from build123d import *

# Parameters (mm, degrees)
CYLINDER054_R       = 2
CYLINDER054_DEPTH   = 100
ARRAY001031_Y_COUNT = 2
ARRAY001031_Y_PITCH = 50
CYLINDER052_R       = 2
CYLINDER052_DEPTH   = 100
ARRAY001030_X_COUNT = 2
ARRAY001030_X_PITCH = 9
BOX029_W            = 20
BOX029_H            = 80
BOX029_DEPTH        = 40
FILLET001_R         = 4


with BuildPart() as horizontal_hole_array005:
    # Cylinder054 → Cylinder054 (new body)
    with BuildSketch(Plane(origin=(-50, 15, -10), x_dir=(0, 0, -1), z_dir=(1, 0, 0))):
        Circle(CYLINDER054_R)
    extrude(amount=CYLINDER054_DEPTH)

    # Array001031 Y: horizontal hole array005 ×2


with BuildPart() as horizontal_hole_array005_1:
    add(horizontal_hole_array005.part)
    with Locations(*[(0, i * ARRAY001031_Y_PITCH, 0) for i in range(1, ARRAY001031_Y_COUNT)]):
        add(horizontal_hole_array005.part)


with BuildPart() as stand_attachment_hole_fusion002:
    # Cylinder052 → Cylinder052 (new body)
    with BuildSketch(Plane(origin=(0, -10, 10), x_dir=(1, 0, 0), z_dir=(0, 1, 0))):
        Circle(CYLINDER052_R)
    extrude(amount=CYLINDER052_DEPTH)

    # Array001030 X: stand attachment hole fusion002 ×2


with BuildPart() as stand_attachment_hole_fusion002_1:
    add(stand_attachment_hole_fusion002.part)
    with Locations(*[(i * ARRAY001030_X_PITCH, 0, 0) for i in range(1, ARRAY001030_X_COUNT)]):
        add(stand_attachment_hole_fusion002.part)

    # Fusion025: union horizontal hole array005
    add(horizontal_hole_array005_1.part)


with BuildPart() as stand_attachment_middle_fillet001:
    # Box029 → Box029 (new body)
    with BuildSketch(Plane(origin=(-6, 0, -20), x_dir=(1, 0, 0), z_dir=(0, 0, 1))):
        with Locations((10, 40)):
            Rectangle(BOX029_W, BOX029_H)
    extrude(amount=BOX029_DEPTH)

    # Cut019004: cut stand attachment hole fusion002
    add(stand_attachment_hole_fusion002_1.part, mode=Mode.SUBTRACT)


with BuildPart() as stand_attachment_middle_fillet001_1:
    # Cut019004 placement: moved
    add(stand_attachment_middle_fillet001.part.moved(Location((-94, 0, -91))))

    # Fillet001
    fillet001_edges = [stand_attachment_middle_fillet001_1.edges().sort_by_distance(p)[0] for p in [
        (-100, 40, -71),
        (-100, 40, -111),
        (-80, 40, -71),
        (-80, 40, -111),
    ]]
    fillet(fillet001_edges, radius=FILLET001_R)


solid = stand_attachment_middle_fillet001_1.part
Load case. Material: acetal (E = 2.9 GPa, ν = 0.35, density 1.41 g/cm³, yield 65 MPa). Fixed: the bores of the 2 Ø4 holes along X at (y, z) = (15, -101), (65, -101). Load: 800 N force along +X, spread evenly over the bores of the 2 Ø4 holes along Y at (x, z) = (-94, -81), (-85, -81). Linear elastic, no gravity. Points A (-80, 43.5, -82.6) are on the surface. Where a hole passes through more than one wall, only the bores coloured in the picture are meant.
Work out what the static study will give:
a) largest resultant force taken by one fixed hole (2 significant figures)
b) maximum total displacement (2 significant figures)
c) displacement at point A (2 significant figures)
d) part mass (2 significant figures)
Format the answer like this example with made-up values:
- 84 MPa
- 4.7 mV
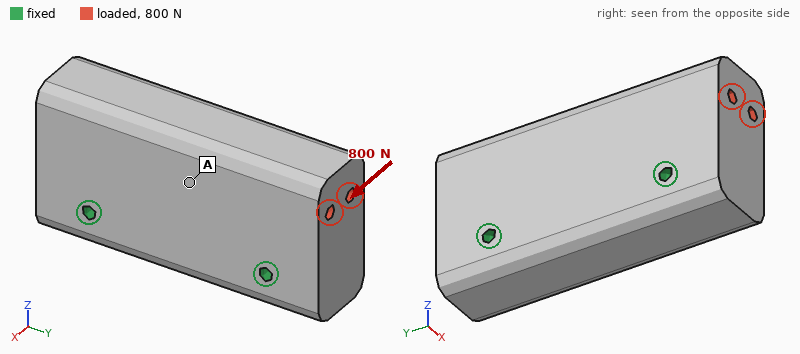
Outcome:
- 400 N
- 84 µm
- 59 µm
- 85 g
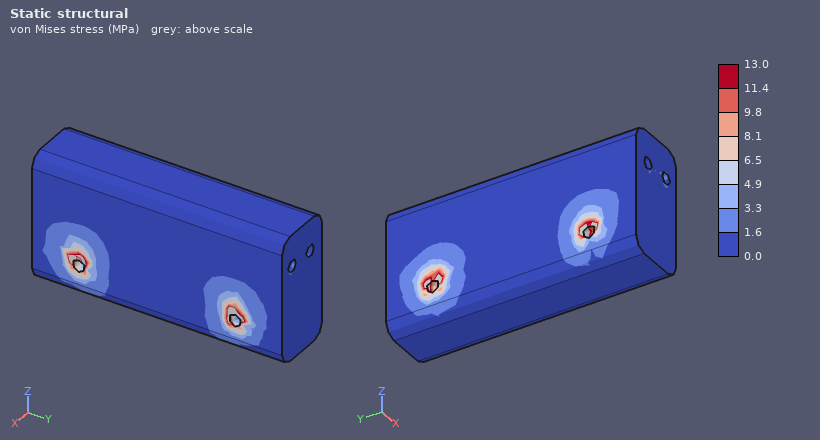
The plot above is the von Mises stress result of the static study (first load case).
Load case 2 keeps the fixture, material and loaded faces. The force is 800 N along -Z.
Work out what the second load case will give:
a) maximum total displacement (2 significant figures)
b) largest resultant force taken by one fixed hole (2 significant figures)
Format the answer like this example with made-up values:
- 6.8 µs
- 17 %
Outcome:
- 10 µm
- 410 N
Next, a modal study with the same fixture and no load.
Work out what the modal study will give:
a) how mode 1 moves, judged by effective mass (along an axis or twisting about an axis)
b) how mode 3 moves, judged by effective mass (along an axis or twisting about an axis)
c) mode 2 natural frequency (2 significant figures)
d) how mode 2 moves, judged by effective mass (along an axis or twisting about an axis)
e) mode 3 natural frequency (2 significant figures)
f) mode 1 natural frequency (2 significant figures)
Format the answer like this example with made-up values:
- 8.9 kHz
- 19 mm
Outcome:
- along X
- along Y
- 4100 Hz
- twisting about Z
- 4800 Hz
- 2700 Hz
